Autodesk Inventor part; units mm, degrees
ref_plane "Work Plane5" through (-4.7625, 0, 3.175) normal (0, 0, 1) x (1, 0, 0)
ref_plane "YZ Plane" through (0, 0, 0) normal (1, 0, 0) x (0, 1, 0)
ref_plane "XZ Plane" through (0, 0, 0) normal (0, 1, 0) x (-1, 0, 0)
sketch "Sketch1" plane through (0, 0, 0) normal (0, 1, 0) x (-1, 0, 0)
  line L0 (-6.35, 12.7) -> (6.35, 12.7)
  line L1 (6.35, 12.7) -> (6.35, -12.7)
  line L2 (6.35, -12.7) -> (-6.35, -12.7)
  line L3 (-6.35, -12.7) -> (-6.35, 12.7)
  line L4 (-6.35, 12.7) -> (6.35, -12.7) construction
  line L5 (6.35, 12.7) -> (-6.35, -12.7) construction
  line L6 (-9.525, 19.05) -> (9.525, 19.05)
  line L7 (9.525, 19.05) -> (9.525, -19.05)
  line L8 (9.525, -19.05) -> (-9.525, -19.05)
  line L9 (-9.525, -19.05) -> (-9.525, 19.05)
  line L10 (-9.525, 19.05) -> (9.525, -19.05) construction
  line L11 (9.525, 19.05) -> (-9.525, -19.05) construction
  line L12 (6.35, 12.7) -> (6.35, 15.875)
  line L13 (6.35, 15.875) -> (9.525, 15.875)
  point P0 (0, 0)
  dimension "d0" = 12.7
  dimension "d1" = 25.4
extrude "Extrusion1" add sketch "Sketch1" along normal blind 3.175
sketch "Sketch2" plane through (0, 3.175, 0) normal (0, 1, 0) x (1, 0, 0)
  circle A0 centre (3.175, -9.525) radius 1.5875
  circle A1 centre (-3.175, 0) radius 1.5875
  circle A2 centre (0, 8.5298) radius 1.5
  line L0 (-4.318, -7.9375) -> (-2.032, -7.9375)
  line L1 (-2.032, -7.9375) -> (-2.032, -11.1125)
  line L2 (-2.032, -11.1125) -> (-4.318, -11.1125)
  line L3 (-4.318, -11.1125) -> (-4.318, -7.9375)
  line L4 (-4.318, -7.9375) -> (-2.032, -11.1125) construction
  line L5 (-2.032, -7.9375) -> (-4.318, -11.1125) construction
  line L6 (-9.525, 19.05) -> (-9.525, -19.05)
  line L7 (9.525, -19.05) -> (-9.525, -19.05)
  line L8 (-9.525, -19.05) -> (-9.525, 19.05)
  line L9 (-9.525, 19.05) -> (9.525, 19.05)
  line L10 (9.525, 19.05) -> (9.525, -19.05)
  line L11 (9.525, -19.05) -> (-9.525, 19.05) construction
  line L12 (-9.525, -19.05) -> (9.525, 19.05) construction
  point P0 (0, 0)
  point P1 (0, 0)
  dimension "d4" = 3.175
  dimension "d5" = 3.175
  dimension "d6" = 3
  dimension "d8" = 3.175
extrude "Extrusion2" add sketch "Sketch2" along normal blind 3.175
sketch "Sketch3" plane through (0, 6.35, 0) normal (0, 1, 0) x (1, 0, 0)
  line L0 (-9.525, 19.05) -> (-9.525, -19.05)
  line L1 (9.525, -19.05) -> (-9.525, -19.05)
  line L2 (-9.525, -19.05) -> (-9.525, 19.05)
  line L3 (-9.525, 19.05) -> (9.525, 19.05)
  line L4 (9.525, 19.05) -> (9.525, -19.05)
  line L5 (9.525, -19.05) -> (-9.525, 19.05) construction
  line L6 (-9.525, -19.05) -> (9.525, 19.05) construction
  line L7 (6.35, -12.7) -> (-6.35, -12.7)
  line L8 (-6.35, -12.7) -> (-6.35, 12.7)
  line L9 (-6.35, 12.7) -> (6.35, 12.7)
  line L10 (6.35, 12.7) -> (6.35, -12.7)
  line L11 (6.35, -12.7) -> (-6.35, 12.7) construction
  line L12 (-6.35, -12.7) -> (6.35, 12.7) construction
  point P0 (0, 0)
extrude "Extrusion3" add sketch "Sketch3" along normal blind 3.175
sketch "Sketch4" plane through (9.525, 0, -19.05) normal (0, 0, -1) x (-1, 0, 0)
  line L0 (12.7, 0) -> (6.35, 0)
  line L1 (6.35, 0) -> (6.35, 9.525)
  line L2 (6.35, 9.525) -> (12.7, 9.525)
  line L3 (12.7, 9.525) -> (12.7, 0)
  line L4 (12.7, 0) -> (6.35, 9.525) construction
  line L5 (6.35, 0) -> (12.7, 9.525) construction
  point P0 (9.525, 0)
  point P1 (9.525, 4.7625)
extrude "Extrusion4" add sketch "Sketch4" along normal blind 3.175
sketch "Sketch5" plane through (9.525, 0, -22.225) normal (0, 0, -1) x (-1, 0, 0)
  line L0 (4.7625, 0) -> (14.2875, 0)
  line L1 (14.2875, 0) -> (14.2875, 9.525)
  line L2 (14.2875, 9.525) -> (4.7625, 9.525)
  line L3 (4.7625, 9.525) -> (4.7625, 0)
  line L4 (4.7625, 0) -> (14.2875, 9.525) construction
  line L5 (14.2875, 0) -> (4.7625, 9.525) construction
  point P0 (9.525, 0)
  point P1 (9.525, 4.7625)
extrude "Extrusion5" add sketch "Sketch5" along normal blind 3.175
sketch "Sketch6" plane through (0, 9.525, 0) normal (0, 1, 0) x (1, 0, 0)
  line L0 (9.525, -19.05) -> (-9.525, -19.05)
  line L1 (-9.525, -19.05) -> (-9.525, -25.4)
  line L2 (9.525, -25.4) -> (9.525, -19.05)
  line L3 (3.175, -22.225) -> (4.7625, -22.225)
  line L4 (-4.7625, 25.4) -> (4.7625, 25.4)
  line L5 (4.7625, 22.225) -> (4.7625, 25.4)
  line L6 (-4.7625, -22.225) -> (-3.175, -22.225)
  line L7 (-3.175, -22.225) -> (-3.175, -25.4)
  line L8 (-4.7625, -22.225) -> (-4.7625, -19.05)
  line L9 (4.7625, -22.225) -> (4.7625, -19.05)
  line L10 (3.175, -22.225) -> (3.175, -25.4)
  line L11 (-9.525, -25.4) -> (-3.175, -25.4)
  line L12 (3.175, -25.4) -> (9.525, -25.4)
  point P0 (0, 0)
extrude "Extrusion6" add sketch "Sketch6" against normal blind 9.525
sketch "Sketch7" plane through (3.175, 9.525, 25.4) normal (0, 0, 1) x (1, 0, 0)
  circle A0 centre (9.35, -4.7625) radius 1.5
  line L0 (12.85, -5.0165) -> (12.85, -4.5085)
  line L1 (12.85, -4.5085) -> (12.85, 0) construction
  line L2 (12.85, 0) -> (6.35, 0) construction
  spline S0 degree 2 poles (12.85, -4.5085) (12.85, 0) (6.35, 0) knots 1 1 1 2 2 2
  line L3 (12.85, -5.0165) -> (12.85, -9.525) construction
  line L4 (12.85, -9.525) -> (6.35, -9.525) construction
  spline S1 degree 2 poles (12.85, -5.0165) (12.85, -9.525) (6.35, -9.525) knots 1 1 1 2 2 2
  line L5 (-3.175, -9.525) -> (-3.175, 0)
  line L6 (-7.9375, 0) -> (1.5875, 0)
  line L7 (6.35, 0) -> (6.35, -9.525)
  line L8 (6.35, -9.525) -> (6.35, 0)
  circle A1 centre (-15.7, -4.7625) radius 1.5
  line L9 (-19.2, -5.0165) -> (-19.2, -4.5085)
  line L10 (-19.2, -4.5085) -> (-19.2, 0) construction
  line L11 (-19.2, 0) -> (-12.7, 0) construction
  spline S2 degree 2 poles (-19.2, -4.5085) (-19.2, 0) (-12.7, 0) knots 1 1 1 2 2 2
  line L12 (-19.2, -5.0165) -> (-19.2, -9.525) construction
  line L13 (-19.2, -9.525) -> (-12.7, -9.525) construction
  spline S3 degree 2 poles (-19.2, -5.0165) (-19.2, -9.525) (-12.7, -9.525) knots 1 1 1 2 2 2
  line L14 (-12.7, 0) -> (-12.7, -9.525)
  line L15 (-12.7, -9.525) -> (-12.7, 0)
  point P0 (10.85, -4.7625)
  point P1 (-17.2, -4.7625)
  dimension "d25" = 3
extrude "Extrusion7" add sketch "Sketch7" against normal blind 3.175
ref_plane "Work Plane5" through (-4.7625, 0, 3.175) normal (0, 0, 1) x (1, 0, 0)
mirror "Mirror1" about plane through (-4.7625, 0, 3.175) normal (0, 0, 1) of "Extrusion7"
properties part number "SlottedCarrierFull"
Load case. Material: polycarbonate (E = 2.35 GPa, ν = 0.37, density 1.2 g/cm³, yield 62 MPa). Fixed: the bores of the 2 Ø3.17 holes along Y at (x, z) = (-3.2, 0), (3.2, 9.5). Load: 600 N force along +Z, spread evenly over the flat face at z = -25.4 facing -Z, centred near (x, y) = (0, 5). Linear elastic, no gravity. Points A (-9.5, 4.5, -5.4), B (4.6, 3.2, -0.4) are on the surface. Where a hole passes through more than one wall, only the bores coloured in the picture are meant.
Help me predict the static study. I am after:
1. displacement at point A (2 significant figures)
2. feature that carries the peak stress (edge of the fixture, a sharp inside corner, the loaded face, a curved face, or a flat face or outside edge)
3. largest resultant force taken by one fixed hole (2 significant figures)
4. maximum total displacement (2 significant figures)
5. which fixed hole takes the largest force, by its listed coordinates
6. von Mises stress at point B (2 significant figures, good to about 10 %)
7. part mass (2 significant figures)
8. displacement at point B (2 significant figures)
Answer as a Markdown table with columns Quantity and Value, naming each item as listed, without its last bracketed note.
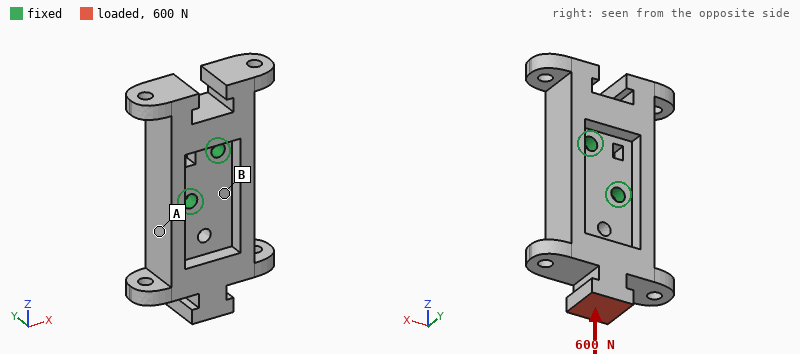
| Quantity | Value |
|---|---|
| displacement at point A | 0.028 mm |
| feature that carries the peak stress | a curved face |
| largest resultant force taken by one fixed hole | 340 N |
| maximum total displacement | 0.14 mm |
| which fixed hole takes the largest force, by its listed coordinates | (-3.2, 0) |
| von Mises stress at point B | 6.2 MPa |
| part mass | 7.8 g |
| displacement at point B | 0.029 mm |
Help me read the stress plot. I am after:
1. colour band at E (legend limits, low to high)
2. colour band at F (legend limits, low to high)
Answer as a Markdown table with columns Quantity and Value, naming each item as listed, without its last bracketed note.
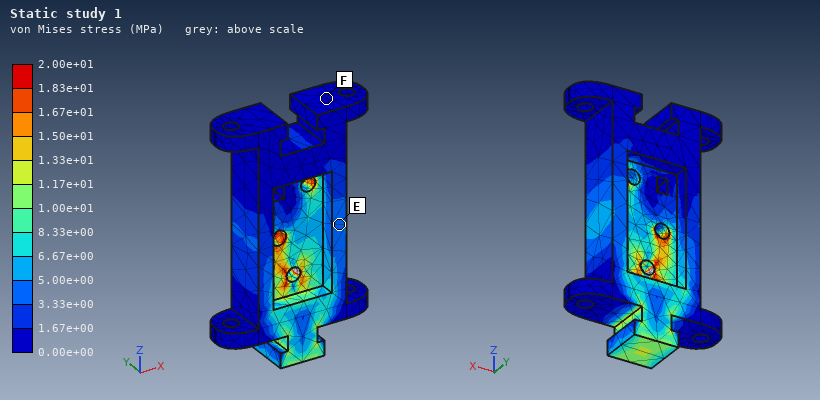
| Quantity | Value |
|---|---|
| colour band at E | 3.33e+00 to 5.00e+00 MPa |
| colour band at F | 0.00e+00 to 1.67e+00 MPa |
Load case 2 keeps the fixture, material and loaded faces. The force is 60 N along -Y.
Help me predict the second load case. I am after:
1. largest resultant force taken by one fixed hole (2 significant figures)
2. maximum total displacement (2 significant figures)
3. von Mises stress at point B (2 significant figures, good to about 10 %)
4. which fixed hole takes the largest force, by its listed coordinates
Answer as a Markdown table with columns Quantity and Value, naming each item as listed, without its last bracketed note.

| Quantity | Value |
|---|---|
| largest resultant force taken by one fixed hole | 120 N |
| maximum total displacement | 0.71 mm |
| von Mises stress at point B | 6.0 MPa |
| which fixed hole takes the largest force, by its listed coordinates | (-3.2, 0) |
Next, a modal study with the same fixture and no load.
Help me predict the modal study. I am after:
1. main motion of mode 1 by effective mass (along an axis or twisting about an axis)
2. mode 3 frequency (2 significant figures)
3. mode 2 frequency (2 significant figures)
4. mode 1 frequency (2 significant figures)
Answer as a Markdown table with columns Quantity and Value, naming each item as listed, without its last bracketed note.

| Quantity | Value |
|---|---|
| main motion of mode 1 by effective mass | along Y |
| mode 3 frequency | 2600 Hz |
| mode 2 frequency | 2500 Hz |
| mode 1 frequency | 1300 Hz |
